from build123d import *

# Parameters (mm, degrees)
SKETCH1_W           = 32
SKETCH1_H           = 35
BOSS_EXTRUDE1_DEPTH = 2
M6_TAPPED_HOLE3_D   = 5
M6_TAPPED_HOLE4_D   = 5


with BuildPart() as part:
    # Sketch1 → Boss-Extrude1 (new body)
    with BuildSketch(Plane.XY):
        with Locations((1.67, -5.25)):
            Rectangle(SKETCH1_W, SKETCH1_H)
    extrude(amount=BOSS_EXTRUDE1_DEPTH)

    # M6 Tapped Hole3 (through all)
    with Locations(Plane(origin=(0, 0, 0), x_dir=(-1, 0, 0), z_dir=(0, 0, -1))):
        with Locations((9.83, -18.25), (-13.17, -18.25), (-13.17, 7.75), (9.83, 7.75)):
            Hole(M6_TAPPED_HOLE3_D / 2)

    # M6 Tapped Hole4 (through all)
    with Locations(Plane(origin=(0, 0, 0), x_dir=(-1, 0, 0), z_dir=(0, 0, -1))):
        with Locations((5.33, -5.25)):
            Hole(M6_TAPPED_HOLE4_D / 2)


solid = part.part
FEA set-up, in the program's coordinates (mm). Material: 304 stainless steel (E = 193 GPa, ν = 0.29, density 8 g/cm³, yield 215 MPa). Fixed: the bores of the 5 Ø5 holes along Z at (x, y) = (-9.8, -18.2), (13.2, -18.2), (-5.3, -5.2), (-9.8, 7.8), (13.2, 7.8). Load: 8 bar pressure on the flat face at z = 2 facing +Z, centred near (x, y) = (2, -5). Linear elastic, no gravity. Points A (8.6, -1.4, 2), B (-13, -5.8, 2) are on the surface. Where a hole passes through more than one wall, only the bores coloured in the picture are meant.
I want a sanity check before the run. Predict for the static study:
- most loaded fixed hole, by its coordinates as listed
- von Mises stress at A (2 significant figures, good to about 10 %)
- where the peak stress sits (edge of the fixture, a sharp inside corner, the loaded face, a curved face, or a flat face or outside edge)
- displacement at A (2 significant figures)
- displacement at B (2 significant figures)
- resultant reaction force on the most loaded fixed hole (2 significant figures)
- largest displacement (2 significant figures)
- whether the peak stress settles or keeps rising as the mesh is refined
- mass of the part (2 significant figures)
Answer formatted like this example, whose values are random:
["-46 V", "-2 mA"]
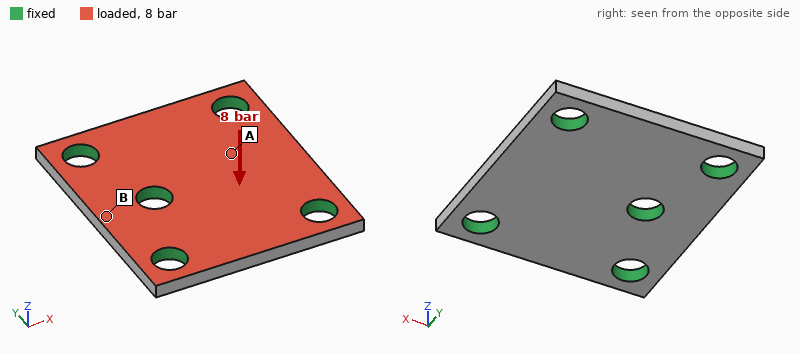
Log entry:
["(-5.3, -5.2)", "16 MPa", "edge of the fixture", "3.4 µm", "1.1 µm", "210 N", "4.5 µm", "keeps rising", "16 g"]
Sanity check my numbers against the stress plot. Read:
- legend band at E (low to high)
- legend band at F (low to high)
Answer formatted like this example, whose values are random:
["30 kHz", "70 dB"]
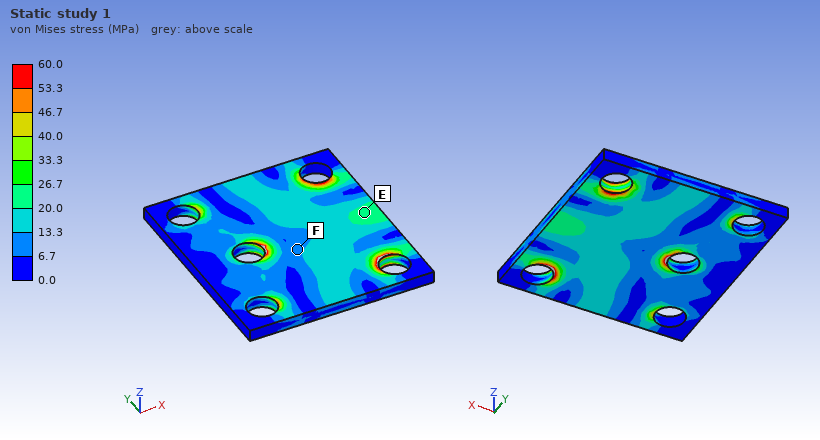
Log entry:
["20.0 to 26.7 MPa", "6.7 to 13.3 MPa"]
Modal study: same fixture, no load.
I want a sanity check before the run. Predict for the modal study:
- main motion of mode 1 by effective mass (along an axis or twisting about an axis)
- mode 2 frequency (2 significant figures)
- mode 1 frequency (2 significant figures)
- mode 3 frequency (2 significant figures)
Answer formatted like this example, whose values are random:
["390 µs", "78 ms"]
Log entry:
["along Z", "26 kHz", "20 kHz", "27 kHz"]
